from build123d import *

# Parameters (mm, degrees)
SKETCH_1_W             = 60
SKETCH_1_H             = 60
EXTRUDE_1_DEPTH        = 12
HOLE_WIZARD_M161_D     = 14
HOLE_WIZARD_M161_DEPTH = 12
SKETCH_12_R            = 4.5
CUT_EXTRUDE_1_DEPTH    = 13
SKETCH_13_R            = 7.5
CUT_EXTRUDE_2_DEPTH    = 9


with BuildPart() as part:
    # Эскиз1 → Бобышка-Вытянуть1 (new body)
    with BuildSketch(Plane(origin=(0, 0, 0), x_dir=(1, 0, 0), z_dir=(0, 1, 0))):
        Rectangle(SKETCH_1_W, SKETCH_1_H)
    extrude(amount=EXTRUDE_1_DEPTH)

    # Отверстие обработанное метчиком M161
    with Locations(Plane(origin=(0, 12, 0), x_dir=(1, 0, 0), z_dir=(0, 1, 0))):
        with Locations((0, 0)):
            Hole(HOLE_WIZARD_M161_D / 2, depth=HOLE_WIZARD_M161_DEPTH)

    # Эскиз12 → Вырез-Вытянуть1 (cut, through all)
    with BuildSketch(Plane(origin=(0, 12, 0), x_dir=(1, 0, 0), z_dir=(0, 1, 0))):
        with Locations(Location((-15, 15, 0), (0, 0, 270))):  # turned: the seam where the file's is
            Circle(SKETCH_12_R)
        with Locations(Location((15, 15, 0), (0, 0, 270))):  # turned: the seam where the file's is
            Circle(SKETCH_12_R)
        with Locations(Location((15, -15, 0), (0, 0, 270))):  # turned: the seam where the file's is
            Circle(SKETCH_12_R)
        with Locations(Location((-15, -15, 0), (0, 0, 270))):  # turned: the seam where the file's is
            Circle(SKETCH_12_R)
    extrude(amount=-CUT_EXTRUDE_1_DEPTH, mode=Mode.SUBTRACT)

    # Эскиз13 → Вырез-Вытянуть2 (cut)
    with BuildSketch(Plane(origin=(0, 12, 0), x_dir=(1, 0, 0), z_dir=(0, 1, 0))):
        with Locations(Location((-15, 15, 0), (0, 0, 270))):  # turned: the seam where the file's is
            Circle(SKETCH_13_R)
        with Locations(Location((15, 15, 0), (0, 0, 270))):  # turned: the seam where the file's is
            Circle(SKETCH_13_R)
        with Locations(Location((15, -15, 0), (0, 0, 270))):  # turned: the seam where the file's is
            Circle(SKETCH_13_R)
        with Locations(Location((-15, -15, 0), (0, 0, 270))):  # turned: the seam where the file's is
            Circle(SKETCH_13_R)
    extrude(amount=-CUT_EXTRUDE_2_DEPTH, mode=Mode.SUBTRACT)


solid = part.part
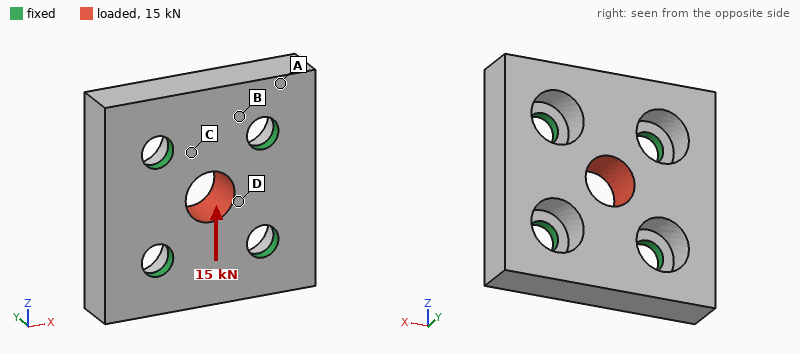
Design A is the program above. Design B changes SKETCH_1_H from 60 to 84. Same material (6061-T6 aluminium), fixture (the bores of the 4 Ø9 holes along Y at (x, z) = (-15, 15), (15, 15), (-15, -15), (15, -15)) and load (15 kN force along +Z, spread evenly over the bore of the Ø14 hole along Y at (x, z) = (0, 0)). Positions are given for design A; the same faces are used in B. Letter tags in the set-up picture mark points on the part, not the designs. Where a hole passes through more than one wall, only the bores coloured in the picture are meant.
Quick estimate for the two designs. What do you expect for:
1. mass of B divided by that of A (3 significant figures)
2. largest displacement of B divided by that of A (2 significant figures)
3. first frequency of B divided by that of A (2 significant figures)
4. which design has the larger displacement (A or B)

1.50
1.2
0.48
B
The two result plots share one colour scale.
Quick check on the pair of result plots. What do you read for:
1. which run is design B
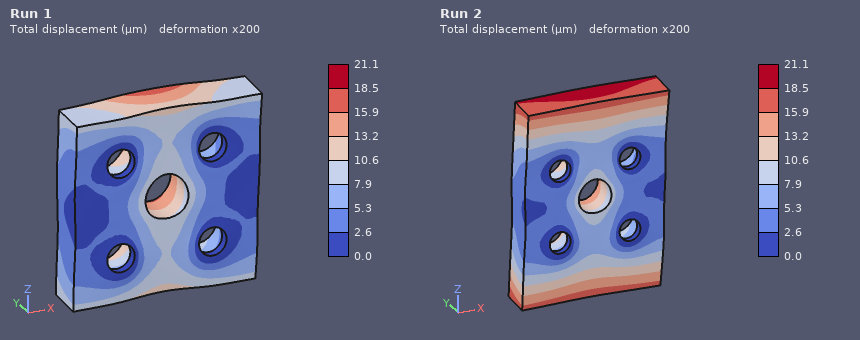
Run 2
